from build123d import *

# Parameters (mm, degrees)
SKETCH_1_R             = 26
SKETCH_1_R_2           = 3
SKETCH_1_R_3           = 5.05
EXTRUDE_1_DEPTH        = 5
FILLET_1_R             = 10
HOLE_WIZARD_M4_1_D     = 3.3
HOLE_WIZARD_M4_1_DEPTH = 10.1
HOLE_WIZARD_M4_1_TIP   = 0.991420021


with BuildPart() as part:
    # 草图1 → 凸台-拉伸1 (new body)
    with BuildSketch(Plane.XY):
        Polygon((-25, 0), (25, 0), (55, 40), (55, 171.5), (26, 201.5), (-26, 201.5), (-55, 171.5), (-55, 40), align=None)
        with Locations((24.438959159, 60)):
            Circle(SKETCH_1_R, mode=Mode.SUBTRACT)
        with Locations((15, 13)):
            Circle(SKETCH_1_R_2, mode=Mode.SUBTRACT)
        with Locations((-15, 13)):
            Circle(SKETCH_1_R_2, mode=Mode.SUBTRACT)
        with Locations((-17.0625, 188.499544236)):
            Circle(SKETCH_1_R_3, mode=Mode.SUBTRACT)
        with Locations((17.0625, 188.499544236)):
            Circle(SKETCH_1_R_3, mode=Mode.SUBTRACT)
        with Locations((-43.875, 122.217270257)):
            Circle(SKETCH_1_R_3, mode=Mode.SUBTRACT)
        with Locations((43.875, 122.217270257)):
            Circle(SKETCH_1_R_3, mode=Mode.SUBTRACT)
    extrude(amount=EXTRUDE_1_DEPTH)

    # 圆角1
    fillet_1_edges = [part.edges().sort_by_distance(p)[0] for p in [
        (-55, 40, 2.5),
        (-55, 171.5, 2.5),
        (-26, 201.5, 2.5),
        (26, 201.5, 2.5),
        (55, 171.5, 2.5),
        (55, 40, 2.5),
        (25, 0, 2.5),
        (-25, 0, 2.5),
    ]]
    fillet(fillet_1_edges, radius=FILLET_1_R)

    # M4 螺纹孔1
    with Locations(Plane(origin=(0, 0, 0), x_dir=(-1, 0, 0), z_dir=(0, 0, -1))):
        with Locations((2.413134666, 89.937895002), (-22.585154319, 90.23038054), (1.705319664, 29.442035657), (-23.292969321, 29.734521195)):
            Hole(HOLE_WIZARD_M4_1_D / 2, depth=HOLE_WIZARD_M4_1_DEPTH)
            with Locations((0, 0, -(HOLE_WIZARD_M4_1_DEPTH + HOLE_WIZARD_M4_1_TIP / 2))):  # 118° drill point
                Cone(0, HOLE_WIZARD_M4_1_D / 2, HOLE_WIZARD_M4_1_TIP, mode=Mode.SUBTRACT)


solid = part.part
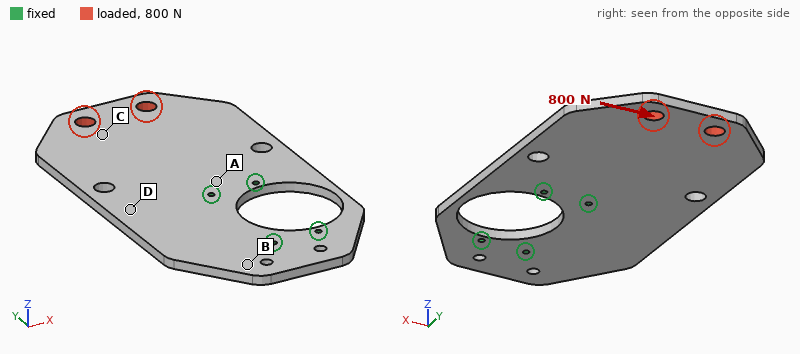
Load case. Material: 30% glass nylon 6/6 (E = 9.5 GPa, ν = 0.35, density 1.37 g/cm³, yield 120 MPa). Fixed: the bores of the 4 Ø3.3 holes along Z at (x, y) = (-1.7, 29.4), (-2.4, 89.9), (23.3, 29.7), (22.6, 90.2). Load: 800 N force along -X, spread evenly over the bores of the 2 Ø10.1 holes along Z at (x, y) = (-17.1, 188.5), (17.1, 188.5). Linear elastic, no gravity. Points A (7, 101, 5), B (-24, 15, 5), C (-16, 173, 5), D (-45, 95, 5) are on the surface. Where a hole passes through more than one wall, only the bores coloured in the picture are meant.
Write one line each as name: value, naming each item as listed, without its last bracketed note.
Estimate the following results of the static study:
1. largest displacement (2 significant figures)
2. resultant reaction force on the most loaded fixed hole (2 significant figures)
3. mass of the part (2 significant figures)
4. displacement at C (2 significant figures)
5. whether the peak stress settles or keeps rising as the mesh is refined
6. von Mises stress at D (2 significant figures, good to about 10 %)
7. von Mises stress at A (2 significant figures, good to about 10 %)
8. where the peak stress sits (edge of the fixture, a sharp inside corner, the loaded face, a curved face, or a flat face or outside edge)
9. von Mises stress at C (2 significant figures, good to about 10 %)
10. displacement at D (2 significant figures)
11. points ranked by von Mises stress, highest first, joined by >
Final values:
largest displacement: 0.30 mm
resultant reaction force on the most loaded fixed hole: 1.3 kN
mass of the part: 120 g
displacement at C: 0.22 mm
whether the peak stress settles or keeps rising as the mesh is refined: keeps rising
von Mises stress at D: 6.2 MPa
von Mises stress at A: 9.4 MPa
where the peak stress sits: edge of the fixture
von Mises stress at C: 4.1 MPa
displacement at D: 0.079 mm
points ranked by von Mises stress, highest first, joined by >: A > D > C > B
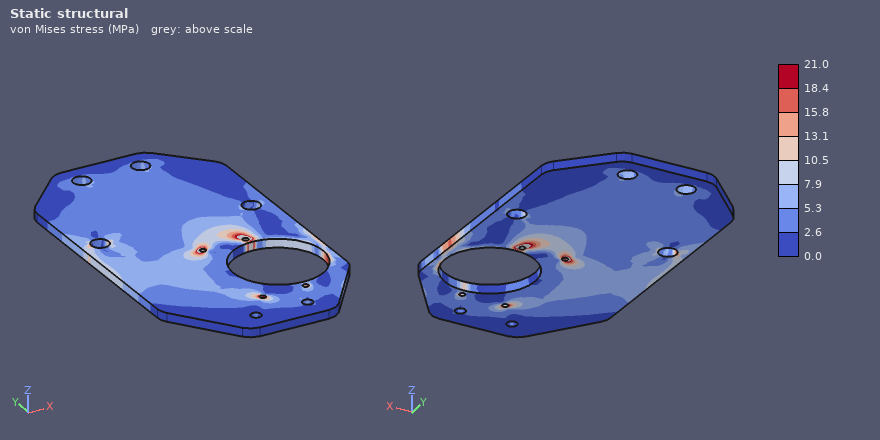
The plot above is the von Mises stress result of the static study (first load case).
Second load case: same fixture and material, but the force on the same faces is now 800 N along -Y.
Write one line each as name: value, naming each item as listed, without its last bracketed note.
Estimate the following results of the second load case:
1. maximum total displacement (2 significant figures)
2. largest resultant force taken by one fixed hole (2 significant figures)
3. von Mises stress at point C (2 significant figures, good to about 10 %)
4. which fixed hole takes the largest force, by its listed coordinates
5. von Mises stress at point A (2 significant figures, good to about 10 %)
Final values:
maximum total displacement: 31 µm
largest resultant force taken by one fixed hole: 390 N
von Mises stress at point C: 2.5 MPa
which fixed hole takes the largest force, by its listed coordinates: (-2.4, 89.9)
von Mises stress at point A: 1.9 MPa
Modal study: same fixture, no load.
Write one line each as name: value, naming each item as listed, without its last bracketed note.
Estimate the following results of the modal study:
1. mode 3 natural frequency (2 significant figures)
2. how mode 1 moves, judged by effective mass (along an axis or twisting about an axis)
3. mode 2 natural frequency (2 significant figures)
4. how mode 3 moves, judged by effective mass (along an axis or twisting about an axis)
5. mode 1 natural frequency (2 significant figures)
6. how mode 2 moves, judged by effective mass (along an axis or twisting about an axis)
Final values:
mode 3 natural frequency: 740 Hz
how mode 1 moves, judged by effective mass: along Z
mode 2 natural frequency: 390 Hz
how mode 3 moves, judged by effective mass: along Z
mode 1 natural frequency: 180 Hz
how mode 2 moves, judged by effective mass: twisting about Y
